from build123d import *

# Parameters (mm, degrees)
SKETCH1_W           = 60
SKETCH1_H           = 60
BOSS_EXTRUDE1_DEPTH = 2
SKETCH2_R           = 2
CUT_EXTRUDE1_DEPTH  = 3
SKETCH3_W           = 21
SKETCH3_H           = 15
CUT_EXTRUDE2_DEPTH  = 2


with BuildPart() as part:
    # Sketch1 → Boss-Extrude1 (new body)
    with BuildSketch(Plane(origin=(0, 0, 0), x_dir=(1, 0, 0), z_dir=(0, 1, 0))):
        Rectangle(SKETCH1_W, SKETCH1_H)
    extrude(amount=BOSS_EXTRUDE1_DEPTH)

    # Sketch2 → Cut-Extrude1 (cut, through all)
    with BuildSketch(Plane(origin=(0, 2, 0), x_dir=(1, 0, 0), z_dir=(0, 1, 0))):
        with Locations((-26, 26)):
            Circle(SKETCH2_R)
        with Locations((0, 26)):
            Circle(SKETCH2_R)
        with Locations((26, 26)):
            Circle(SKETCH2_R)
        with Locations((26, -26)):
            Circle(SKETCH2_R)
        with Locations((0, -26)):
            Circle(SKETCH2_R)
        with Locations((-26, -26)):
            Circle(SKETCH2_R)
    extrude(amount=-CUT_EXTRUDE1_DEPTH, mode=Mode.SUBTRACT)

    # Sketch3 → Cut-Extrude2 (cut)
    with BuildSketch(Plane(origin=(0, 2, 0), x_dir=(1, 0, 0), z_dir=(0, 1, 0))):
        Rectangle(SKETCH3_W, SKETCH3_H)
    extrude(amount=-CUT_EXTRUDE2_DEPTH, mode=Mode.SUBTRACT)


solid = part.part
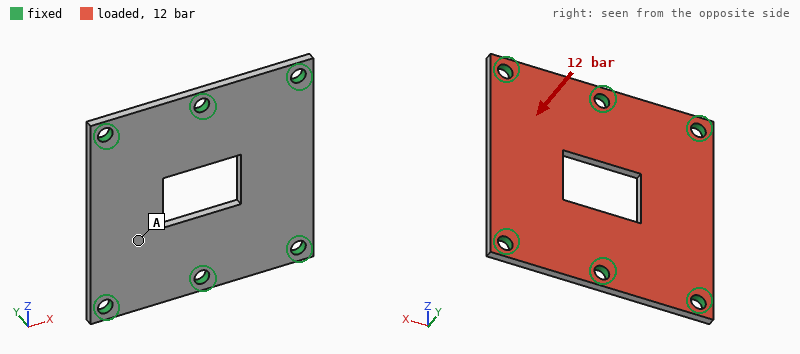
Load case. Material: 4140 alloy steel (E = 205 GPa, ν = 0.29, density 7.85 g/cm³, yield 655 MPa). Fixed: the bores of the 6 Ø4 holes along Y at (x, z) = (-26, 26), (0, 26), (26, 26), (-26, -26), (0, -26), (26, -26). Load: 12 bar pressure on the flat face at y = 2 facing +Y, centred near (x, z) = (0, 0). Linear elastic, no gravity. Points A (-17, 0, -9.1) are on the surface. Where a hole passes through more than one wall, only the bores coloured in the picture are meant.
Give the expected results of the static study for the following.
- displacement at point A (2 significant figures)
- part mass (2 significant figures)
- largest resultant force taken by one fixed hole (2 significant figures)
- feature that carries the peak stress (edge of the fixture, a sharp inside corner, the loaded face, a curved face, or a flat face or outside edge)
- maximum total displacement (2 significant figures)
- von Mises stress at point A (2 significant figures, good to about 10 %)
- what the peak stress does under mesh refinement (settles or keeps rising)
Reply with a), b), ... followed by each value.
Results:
a) 0.13 mm
b) 50 g
c) 820 N
d) edge of the fixture
e) 0.18 mm
f) 110 MPa
g) keeps rising
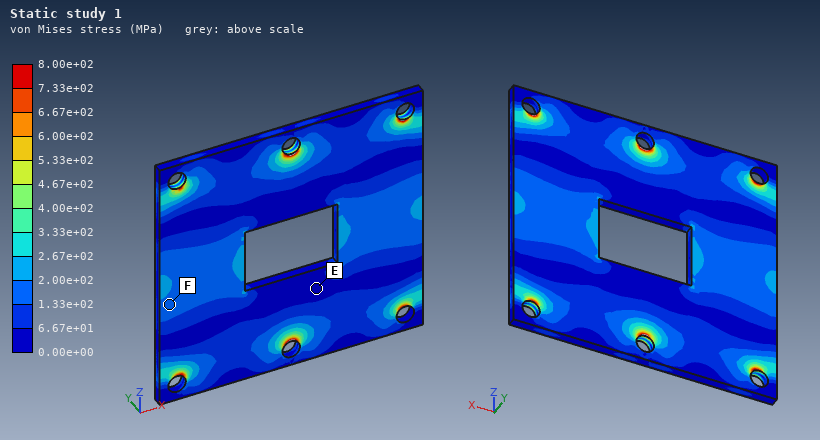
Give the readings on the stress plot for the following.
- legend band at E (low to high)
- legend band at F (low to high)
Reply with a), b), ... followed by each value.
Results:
a) 0.00e+00 to 6.67e+01 MPa
b) 1.33e+02 to 2.00e+02 MPa
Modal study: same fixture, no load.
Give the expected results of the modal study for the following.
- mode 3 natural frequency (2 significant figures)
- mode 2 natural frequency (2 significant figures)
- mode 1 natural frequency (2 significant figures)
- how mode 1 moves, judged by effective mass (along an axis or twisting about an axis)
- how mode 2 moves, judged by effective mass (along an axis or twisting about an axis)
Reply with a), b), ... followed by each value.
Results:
a) 7300 Hz
b) 4500 Hz
c) 4000 Hz
d) along Y
e) twisting about Z
